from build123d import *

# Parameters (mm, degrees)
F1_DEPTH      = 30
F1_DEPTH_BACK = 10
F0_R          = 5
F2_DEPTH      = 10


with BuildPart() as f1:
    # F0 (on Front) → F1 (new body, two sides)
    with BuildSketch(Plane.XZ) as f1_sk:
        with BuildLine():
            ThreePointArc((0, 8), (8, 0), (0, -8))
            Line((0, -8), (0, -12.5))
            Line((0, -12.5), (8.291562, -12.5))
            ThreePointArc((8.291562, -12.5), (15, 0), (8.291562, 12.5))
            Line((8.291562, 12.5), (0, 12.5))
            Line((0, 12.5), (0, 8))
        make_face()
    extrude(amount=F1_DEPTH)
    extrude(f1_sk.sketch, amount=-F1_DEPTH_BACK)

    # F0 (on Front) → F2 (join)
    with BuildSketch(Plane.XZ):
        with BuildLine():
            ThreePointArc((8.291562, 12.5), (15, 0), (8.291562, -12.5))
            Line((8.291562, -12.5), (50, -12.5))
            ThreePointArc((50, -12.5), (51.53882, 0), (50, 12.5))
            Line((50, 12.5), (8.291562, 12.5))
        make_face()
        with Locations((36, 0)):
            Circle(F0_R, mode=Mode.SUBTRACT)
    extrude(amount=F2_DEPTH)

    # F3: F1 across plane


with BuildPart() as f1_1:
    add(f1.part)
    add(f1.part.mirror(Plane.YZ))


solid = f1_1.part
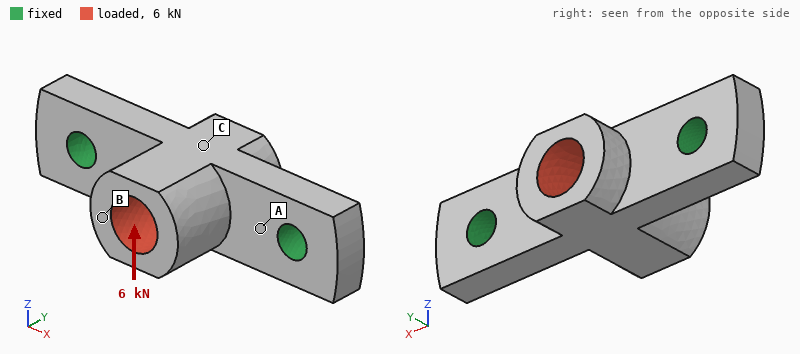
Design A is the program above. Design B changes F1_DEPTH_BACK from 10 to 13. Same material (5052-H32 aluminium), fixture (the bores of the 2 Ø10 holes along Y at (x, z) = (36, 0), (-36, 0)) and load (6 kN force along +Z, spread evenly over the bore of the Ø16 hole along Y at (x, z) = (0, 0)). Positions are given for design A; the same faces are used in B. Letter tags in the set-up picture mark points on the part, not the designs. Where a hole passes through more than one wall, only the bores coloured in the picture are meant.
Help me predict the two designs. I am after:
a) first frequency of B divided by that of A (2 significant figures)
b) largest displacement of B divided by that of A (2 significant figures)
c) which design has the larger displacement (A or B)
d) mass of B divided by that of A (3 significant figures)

0.96
0.82
A
1.04
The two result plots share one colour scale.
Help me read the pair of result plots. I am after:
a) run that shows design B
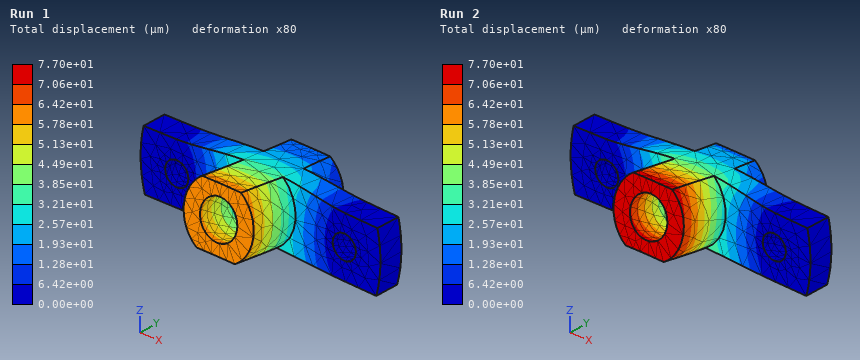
Run 1
